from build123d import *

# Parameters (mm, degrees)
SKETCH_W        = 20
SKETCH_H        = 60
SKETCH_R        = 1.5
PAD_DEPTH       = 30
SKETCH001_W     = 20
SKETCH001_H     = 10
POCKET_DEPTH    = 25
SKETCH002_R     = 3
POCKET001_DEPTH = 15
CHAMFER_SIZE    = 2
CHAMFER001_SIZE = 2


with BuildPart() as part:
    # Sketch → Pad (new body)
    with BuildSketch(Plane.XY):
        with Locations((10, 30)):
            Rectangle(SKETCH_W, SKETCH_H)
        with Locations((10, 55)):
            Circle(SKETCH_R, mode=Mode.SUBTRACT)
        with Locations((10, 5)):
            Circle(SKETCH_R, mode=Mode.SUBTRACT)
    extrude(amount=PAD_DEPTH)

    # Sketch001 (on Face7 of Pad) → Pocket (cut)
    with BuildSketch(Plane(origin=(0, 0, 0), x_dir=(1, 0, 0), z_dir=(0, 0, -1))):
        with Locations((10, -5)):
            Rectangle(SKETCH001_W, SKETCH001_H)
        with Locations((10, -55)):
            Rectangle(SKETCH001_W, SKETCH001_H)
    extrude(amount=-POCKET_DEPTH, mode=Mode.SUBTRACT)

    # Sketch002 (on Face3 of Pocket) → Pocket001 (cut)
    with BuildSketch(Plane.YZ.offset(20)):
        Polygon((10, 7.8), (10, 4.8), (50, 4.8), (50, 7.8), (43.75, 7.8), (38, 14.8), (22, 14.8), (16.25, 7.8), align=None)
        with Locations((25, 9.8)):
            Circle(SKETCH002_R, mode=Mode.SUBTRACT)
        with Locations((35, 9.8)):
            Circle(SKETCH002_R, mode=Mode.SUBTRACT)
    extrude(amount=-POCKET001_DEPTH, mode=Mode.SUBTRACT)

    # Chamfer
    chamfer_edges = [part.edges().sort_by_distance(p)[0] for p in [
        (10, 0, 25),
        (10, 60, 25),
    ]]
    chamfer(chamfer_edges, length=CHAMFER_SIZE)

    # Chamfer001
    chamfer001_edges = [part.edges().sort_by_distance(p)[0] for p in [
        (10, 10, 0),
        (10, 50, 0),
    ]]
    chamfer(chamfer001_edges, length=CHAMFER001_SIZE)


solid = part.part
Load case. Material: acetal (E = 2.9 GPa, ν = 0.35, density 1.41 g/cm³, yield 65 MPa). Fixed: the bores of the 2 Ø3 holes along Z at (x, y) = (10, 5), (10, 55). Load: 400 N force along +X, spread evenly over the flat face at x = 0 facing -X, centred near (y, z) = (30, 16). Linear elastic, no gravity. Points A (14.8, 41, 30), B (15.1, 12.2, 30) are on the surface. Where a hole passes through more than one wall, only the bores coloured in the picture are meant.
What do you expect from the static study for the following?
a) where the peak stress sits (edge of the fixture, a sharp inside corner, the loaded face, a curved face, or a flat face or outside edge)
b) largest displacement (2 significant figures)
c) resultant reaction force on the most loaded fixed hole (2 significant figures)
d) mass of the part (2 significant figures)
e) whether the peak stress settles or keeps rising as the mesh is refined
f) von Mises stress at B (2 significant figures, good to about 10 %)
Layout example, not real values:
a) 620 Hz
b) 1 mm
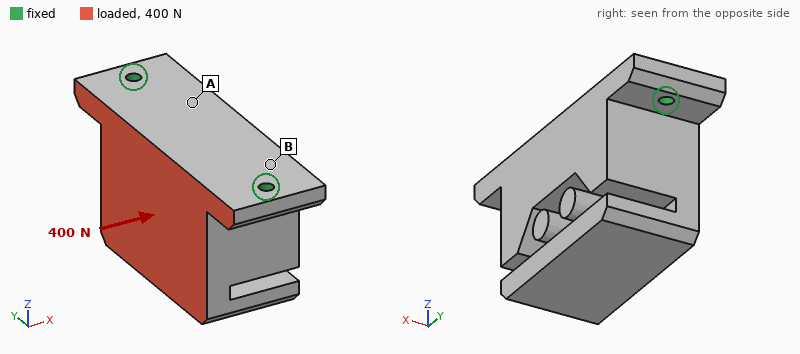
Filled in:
a) edge of the fixture
b) 0.74 mm
c) 200 N
d) 32 g
e) keeps rising
f) 7.7 MPa
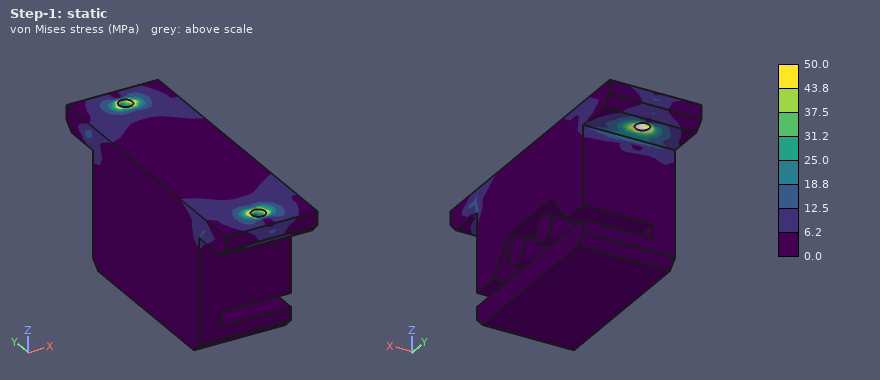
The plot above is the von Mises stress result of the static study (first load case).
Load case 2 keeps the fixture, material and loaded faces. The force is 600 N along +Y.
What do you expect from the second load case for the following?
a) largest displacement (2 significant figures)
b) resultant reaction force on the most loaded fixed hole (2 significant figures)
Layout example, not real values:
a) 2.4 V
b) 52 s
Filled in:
a) 84 µm
b) 360 N
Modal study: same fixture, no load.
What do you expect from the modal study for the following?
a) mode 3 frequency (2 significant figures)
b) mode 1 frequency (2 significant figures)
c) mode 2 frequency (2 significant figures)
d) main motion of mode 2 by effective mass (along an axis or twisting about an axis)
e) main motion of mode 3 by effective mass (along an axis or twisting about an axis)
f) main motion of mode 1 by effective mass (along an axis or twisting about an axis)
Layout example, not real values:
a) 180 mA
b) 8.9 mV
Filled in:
a) 2600 Hz
b) 820 Hz
c) 2100 Hz
d) along Z
e) along Y
f) along X
